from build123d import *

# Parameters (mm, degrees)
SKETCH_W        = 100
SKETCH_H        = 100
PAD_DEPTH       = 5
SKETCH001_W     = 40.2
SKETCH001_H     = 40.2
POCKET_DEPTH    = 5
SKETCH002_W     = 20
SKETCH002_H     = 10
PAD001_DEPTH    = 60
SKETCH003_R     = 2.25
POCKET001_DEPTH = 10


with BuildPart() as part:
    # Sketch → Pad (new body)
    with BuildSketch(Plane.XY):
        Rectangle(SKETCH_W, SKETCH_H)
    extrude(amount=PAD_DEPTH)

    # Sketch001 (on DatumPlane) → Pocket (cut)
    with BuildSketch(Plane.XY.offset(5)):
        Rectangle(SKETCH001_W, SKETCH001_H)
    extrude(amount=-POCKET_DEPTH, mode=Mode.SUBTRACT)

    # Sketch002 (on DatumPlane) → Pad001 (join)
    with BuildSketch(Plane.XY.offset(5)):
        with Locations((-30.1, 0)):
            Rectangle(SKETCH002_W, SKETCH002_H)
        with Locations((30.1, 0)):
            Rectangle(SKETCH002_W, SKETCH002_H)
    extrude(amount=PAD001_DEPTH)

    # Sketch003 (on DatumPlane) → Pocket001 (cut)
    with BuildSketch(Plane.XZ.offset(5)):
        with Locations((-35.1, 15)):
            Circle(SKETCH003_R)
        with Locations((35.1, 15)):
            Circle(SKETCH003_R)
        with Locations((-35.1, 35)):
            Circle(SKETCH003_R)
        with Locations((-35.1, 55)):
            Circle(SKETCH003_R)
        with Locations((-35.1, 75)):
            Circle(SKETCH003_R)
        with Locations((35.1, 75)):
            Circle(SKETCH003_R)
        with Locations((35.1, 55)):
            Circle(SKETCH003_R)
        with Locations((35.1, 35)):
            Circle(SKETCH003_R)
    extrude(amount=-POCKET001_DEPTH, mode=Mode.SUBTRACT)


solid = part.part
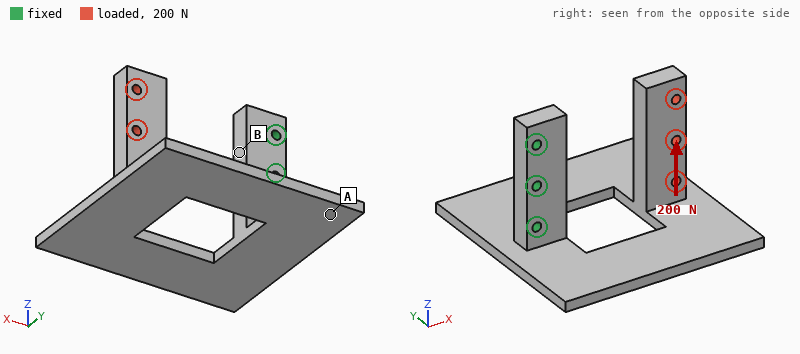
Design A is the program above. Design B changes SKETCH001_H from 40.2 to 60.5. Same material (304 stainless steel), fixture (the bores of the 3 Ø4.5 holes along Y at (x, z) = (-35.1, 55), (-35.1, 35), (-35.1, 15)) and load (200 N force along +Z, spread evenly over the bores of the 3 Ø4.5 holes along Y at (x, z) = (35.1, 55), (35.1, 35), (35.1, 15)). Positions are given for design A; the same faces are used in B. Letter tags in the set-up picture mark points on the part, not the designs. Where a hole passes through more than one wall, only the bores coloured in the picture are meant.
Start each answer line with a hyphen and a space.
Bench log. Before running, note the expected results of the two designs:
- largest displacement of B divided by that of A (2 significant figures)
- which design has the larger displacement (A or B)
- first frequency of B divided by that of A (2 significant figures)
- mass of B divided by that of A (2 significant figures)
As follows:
- 1.5
- B
- 0.84
- 0.94
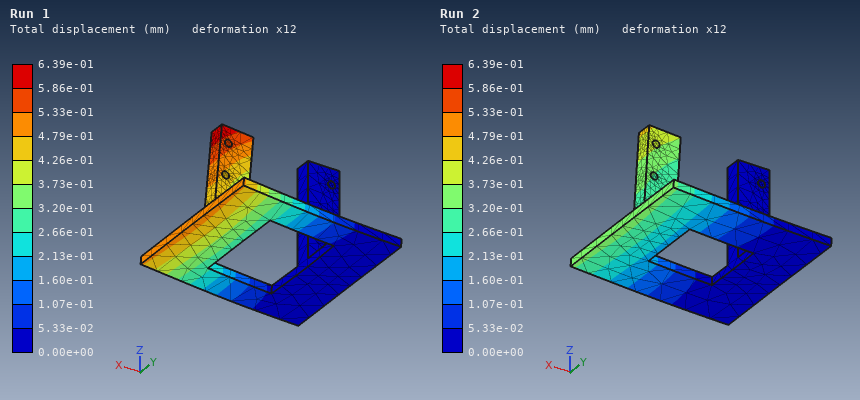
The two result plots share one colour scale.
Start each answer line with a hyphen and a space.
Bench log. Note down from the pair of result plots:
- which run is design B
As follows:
- Run 1
